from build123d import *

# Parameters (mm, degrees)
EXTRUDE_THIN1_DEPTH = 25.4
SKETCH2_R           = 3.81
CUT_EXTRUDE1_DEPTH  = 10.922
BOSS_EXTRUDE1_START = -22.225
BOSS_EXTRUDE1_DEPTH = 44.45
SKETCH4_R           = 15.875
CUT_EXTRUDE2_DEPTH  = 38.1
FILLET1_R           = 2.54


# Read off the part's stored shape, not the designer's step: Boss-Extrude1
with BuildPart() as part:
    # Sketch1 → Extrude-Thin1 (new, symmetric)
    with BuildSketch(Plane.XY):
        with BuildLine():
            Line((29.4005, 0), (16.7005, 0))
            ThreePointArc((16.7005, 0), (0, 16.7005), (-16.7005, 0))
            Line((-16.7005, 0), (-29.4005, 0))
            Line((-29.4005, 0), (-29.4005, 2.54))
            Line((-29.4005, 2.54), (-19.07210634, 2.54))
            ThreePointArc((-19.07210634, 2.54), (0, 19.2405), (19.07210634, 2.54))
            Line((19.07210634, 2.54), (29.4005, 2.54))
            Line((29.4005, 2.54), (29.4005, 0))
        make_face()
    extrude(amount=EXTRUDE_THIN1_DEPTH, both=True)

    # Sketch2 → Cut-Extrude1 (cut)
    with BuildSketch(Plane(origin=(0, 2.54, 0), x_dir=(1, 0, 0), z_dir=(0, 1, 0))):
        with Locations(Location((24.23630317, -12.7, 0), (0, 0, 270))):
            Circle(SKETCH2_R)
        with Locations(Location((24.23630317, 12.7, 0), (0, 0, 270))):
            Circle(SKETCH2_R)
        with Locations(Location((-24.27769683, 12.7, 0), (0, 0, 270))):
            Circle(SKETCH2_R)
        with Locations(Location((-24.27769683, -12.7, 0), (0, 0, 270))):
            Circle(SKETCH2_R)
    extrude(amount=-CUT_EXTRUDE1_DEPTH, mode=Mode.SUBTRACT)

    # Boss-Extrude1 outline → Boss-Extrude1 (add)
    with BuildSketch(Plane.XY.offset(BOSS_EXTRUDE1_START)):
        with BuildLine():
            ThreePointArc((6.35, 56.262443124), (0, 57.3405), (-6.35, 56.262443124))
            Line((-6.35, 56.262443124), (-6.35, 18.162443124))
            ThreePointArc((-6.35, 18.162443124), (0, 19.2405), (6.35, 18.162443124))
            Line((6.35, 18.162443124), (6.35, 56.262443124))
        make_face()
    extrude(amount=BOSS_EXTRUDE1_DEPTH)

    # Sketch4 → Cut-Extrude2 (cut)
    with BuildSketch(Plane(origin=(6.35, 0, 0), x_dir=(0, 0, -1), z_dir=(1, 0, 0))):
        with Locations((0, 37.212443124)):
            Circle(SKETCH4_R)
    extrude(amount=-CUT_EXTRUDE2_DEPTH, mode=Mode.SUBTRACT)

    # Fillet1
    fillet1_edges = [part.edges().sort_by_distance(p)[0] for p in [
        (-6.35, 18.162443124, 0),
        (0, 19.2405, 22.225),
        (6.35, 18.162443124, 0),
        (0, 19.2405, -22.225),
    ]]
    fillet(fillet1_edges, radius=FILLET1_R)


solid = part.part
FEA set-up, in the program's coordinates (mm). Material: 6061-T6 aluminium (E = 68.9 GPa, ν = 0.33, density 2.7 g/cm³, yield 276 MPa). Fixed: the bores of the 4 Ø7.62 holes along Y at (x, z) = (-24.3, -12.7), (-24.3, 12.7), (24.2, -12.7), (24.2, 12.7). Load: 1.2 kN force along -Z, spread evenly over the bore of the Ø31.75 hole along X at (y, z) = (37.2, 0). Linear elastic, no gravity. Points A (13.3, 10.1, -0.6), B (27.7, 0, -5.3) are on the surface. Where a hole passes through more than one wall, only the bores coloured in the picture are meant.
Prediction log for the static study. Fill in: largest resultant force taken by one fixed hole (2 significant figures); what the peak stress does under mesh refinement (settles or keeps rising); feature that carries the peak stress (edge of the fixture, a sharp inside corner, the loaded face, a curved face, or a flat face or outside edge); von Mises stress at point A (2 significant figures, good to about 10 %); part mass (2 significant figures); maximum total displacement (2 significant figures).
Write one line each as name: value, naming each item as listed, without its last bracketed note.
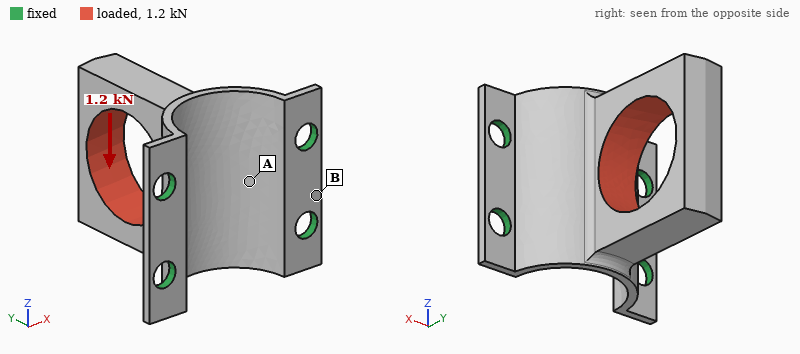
largest resultant force taken by one fixed hole: 980 N
what the peak stress does under mesh refinement: keeps rising
feature that carries the peak stress: edge of the fixture
von Mises stress at point A: 23 MPa
part mass: 57 g
maximum total displacement: 0.10 mm
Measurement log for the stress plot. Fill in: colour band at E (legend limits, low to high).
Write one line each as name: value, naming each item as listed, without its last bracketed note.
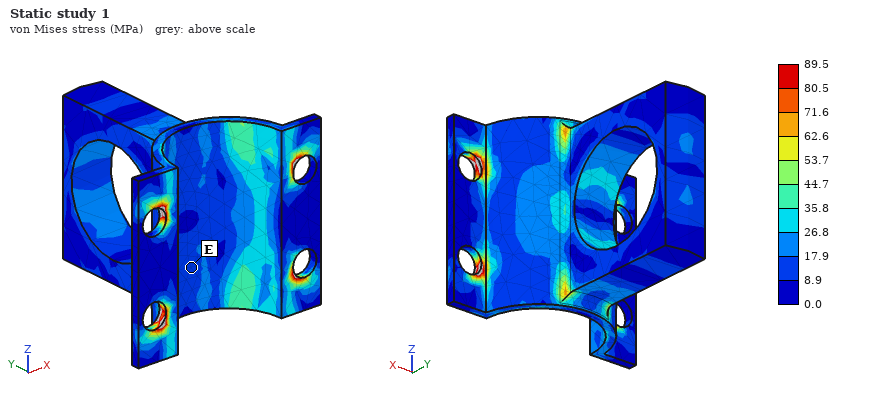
colour band at E: 8.9 to 17.9 MPa
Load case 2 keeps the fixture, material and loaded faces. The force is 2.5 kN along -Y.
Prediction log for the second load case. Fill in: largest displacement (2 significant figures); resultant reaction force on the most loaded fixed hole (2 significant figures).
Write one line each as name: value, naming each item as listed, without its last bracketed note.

largest displacement: 37 µm
resultant reaction force on the most loaded fixed hole: 790 N
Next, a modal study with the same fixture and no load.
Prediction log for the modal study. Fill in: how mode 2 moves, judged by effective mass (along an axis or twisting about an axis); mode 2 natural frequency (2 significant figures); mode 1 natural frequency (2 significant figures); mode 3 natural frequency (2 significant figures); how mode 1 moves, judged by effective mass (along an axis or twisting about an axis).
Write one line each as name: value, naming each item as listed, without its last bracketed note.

how mode 2 moves, judged by effective mass: along Z
mode 2 natural frequency: 3300 Hz
mode 1 natural frequency: 2600 Hz
mode 3 natural frequency: 6200 Hz
how mode 1 moves, judged by effective mass: along X
